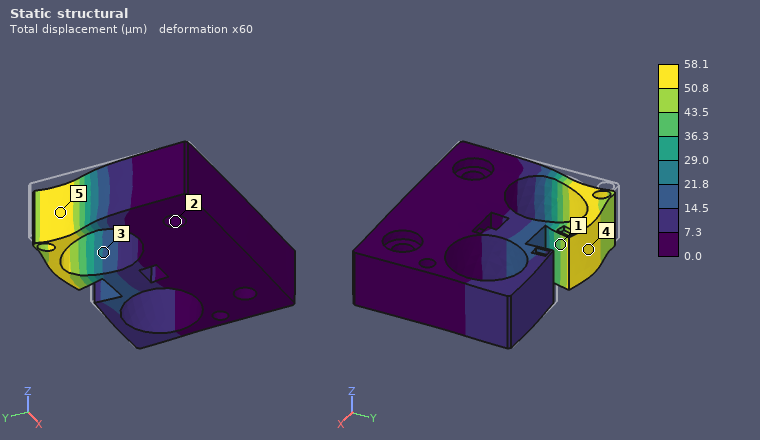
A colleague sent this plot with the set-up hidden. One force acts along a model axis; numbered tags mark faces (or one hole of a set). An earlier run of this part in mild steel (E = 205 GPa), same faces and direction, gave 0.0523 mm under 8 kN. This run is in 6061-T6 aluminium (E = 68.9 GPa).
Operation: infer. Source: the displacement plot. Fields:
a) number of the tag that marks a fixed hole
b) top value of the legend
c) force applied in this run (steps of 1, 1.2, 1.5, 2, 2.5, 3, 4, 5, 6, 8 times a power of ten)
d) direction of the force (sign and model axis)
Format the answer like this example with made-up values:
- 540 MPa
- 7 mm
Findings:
- 2
- 58.1 µm
- 3 kN
- +X
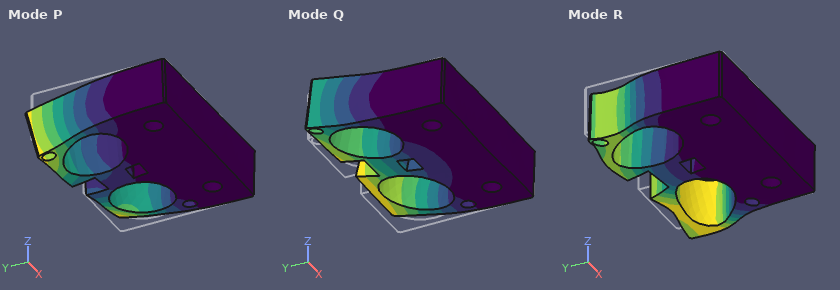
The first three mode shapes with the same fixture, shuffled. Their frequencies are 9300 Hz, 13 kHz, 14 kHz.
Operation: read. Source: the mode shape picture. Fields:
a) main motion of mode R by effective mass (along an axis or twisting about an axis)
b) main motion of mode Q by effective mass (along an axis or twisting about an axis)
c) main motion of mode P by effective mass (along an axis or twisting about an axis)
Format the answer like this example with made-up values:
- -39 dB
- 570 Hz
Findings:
- along X
- along Z
- twisting about Y
